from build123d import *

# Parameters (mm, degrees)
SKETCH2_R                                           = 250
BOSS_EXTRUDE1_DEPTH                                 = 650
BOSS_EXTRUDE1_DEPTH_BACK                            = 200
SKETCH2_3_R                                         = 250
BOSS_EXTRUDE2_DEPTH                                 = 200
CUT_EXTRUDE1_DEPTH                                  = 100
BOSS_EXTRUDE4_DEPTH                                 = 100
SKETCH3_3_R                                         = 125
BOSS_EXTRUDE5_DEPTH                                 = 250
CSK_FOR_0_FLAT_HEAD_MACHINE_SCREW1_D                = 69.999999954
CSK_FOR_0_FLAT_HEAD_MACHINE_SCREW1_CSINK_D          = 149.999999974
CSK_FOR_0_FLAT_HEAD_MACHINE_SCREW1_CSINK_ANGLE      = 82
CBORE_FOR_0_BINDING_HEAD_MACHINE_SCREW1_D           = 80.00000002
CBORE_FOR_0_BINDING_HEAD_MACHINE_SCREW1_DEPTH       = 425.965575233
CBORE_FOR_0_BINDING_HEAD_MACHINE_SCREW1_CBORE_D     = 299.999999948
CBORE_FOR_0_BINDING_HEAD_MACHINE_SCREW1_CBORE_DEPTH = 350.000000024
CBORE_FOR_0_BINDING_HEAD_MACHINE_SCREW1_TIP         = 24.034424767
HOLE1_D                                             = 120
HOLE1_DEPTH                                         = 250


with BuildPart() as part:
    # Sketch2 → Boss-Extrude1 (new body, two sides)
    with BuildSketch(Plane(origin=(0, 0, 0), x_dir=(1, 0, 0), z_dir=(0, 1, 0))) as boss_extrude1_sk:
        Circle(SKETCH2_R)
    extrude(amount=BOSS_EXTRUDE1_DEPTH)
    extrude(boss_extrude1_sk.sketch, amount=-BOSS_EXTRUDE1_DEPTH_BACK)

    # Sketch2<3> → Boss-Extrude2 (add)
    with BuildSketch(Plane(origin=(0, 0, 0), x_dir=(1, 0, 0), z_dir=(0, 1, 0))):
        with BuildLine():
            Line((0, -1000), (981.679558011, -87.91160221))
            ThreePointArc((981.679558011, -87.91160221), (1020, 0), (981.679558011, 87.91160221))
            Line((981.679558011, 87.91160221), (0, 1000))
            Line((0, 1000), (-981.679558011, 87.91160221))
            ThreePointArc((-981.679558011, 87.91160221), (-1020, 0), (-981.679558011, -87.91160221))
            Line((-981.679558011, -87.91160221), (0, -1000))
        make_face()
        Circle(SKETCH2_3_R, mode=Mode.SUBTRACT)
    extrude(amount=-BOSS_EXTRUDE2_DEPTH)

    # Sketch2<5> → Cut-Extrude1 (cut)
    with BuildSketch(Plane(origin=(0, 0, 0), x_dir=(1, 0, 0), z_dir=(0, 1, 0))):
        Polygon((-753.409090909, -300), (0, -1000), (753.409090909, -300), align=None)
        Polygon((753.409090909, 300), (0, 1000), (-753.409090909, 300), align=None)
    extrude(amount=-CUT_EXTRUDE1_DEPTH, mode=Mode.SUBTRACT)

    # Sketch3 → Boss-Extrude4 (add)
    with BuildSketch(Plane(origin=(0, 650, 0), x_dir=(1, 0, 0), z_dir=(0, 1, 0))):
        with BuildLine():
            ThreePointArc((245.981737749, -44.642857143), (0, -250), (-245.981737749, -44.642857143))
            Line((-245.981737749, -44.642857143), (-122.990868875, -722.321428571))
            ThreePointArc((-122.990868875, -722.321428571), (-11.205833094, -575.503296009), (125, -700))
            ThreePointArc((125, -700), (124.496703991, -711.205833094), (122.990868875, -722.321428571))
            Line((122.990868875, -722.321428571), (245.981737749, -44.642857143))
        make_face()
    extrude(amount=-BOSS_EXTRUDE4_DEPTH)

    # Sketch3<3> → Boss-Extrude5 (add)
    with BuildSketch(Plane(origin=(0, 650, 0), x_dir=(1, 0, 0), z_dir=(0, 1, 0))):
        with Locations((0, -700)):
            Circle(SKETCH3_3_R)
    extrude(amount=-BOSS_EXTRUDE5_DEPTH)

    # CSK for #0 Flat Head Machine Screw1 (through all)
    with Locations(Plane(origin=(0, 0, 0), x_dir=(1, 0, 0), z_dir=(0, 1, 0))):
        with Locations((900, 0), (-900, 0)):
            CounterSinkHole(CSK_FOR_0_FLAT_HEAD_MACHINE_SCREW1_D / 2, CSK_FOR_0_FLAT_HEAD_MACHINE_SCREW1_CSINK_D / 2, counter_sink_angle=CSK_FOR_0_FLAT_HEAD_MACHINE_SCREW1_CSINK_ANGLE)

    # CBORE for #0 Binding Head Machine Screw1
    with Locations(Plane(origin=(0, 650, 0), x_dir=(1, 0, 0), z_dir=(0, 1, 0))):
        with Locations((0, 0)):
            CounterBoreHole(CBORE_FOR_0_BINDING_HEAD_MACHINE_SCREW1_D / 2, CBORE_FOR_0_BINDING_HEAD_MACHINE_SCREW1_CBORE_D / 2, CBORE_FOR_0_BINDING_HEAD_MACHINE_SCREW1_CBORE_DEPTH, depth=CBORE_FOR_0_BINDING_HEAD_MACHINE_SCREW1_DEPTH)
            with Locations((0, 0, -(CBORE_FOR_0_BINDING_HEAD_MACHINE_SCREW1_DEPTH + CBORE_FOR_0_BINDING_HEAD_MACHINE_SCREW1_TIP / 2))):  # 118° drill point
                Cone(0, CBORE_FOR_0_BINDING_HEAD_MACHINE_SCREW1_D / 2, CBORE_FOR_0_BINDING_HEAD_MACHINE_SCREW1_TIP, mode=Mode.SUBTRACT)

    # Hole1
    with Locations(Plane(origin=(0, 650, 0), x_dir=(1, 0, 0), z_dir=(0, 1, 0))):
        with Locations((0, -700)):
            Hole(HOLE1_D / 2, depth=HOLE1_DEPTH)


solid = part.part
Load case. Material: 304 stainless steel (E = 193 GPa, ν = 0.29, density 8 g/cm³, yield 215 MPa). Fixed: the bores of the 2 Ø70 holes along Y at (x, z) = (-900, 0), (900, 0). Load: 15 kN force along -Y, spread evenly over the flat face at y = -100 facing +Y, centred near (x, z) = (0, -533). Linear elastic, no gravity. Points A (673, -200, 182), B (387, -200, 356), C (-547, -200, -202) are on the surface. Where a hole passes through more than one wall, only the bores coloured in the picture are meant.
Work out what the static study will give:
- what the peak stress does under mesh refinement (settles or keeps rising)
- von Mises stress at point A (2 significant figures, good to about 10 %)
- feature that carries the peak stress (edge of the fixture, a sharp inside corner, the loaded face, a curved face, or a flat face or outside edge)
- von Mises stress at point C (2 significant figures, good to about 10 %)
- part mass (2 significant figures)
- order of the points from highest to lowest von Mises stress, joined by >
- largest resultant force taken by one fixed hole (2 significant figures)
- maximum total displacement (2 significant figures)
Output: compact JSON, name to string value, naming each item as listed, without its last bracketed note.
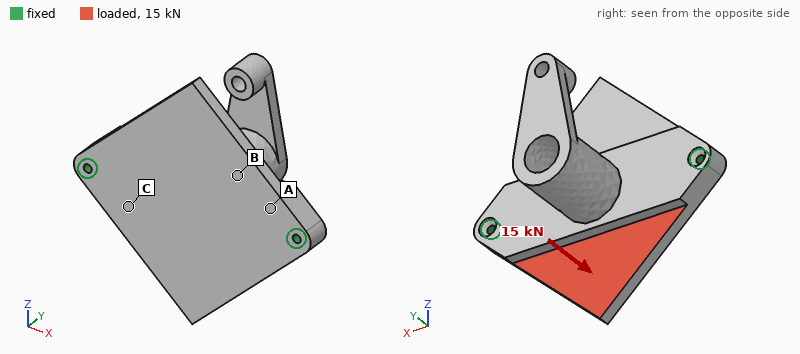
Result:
{"what the peak stress does under mesh refinement": "keeps rising", "von Mises stress at point A": "0.65 MPa", "feature that carries the peak stress": "edge of the fixture", "von Mises stress at point C": "0.90 MPa", "part mass": "3600 kg", "order of the points from highest to lowest von Mises stress, joined by >": "C > A > B", "largest resultant force taken by one fixed hole": "7.7 kN", "maximum total displacement": "71 µm"}
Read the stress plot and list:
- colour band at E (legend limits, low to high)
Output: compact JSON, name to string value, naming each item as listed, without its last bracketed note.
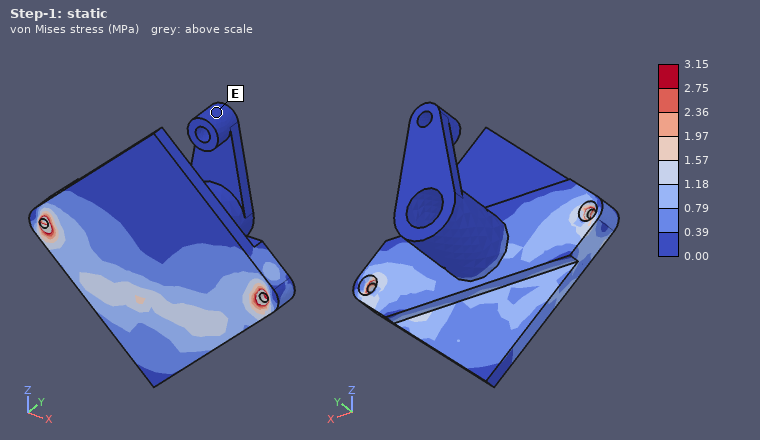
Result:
{"colour band at E": "0.00 to 0.39 MPa"}
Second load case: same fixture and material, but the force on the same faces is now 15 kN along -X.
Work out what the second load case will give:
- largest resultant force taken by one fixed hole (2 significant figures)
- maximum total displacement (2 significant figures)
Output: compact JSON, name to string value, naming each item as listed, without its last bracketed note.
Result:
{"largest resultant force taken by one fixed hole": "8.7 kN", "maximum total displacement": "1.7 µm"}
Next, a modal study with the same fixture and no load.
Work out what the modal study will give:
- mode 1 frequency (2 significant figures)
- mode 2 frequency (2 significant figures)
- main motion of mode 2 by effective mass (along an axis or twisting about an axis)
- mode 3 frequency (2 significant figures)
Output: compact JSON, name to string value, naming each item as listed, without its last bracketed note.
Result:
{"mode 1 frequency": "91 Hz", "mode 2 frequency": "140 Hz", "main motion of mode 2 by effective mass": "along Y", "mode 3 frequency": "180 Hz"}
